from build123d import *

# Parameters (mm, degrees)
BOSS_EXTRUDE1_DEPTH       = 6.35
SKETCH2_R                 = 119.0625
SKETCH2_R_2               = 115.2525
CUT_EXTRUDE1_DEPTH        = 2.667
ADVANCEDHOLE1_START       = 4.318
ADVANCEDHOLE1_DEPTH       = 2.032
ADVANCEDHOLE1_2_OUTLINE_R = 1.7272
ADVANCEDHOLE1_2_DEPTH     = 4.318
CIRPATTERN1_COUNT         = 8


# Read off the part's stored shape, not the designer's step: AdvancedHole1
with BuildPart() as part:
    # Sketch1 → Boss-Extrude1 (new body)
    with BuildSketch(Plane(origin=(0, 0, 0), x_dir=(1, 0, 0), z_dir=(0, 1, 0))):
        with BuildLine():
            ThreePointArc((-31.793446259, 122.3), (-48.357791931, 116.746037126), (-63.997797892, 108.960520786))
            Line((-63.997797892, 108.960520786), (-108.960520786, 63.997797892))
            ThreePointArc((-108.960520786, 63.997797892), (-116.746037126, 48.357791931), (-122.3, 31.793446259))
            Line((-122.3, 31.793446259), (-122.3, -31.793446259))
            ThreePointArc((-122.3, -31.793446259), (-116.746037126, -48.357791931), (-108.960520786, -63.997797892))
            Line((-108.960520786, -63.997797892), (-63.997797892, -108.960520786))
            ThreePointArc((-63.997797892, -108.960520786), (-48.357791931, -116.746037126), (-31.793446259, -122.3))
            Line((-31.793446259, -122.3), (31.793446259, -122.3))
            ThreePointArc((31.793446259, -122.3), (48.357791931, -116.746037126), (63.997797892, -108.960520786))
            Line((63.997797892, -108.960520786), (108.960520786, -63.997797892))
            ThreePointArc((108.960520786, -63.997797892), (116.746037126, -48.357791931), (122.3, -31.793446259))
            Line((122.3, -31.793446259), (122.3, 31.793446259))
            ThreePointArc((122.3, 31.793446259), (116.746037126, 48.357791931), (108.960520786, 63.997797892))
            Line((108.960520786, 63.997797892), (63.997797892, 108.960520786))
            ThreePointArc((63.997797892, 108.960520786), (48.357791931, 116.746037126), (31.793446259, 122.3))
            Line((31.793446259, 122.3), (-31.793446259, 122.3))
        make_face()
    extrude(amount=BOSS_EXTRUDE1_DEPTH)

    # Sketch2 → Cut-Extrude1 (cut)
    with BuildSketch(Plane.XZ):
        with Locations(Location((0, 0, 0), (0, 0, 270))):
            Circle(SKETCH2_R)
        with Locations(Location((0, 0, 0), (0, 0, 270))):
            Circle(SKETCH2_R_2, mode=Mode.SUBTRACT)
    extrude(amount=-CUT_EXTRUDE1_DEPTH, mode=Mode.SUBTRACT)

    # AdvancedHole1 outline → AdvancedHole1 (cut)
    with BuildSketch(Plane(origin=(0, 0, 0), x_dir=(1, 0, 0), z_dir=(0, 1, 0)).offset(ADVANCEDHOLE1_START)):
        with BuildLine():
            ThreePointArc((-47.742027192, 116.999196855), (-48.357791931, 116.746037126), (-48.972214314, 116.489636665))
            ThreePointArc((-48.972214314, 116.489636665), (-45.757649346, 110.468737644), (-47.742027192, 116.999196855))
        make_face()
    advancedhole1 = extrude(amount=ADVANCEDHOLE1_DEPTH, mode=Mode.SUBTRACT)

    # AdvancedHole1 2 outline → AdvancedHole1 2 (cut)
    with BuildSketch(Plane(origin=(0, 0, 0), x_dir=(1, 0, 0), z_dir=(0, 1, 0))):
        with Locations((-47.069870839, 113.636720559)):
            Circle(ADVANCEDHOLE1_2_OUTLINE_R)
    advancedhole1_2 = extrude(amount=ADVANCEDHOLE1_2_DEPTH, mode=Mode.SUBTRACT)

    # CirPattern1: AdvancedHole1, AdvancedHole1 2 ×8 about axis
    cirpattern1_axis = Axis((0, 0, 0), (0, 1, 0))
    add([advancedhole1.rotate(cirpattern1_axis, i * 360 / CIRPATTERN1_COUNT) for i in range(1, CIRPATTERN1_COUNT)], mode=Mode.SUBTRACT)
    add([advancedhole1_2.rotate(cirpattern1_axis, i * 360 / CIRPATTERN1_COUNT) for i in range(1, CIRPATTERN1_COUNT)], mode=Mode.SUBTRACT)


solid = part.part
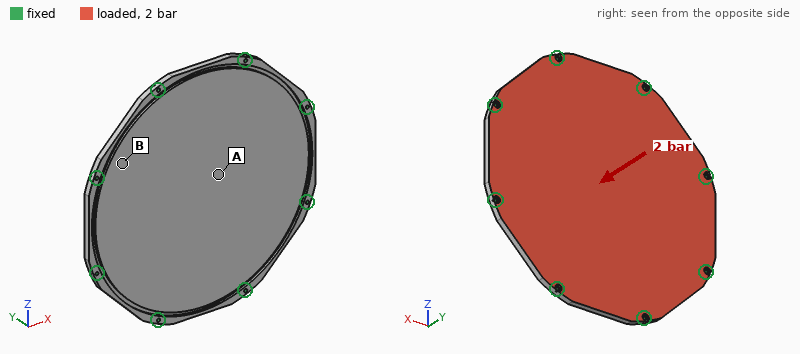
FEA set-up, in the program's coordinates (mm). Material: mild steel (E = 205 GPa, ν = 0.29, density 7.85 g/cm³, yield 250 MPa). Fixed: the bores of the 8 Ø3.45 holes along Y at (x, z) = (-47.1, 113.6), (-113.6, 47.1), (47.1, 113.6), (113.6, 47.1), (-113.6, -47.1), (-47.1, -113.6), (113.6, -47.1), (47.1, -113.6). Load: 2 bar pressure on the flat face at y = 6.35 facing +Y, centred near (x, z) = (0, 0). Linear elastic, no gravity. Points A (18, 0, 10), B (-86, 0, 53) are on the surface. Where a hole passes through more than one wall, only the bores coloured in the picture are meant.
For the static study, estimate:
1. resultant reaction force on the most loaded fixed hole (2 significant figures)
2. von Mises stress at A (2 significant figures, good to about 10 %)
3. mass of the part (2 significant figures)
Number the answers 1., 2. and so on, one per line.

1. 1.2 kN
2. 65 MPa
3. 2.4 kg
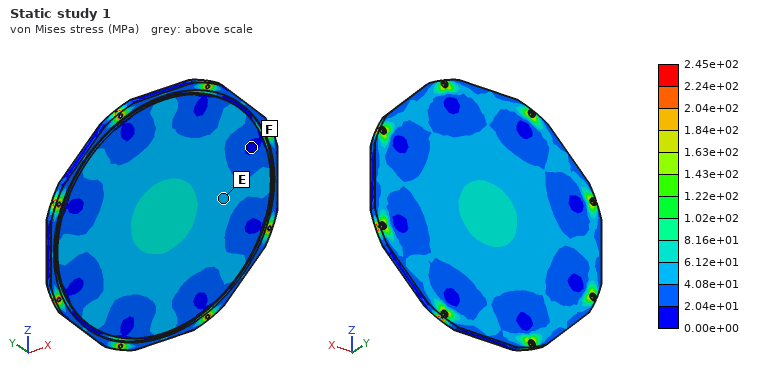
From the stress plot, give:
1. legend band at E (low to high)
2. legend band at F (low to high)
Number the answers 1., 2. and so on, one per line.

1. 4.08e+01 to 6.12e+01 MPa
2. 0.00e+00 to 2.04e+01 MPa
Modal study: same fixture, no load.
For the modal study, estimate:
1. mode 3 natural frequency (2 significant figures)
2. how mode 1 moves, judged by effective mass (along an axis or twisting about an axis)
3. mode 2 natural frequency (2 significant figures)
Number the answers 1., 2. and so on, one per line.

1. 1500 Hz
2. along Y
3. 1500 Hz
